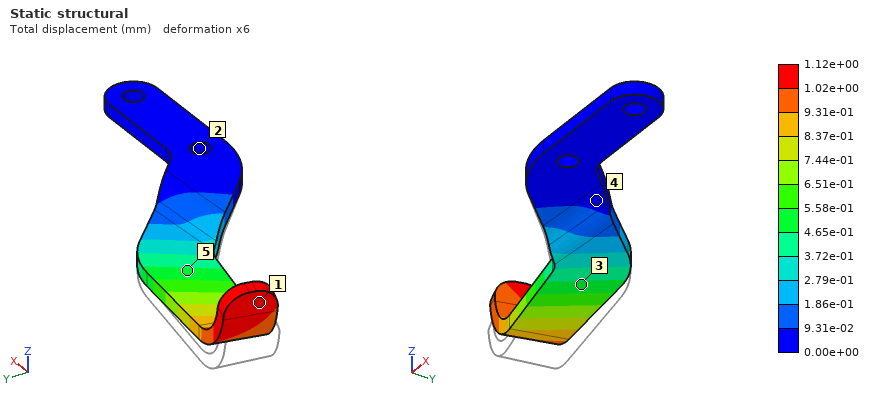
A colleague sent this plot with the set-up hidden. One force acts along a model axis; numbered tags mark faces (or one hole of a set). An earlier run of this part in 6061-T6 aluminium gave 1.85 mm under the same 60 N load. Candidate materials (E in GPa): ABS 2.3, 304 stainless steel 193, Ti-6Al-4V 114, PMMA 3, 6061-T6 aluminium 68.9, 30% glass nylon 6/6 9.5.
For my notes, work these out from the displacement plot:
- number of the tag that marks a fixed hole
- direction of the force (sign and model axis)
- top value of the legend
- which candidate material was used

2
+Z
1.12e+00 mm
Ti-6Al-4V
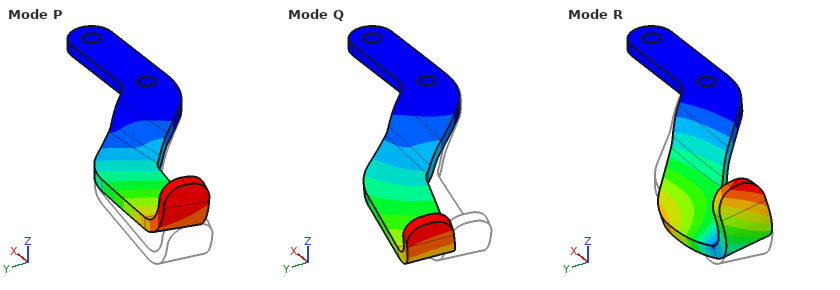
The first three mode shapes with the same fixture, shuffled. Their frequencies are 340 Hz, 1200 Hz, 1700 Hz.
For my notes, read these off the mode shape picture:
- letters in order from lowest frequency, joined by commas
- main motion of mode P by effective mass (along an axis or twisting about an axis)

P, Q, R
along Z
